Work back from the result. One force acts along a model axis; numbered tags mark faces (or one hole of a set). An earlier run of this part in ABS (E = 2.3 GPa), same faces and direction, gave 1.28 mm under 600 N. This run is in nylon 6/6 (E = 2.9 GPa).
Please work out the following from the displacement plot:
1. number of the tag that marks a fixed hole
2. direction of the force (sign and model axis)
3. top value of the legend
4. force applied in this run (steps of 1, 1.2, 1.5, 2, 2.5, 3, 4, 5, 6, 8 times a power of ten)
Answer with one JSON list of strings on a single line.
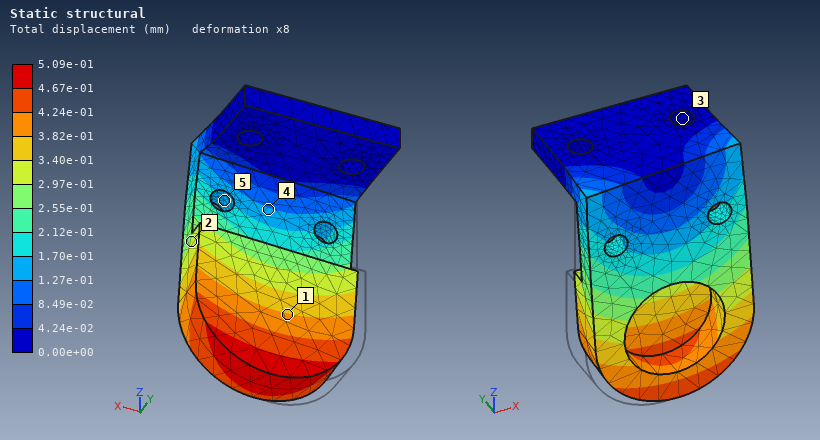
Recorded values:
["3", "+X", "5.09e-01 mm", "300 N"]
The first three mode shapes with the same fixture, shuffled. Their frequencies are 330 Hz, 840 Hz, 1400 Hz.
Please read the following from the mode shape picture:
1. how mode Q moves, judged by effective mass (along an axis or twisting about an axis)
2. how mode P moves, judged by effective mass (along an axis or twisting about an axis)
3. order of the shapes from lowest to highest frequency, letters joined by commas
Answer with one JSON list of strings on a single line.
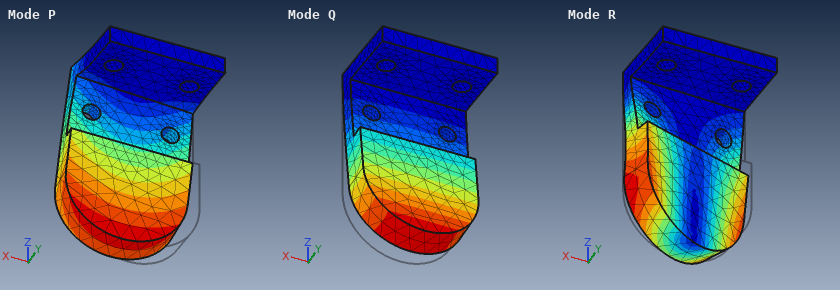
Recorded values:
["along Y", "along X", "Q, P, R"]
